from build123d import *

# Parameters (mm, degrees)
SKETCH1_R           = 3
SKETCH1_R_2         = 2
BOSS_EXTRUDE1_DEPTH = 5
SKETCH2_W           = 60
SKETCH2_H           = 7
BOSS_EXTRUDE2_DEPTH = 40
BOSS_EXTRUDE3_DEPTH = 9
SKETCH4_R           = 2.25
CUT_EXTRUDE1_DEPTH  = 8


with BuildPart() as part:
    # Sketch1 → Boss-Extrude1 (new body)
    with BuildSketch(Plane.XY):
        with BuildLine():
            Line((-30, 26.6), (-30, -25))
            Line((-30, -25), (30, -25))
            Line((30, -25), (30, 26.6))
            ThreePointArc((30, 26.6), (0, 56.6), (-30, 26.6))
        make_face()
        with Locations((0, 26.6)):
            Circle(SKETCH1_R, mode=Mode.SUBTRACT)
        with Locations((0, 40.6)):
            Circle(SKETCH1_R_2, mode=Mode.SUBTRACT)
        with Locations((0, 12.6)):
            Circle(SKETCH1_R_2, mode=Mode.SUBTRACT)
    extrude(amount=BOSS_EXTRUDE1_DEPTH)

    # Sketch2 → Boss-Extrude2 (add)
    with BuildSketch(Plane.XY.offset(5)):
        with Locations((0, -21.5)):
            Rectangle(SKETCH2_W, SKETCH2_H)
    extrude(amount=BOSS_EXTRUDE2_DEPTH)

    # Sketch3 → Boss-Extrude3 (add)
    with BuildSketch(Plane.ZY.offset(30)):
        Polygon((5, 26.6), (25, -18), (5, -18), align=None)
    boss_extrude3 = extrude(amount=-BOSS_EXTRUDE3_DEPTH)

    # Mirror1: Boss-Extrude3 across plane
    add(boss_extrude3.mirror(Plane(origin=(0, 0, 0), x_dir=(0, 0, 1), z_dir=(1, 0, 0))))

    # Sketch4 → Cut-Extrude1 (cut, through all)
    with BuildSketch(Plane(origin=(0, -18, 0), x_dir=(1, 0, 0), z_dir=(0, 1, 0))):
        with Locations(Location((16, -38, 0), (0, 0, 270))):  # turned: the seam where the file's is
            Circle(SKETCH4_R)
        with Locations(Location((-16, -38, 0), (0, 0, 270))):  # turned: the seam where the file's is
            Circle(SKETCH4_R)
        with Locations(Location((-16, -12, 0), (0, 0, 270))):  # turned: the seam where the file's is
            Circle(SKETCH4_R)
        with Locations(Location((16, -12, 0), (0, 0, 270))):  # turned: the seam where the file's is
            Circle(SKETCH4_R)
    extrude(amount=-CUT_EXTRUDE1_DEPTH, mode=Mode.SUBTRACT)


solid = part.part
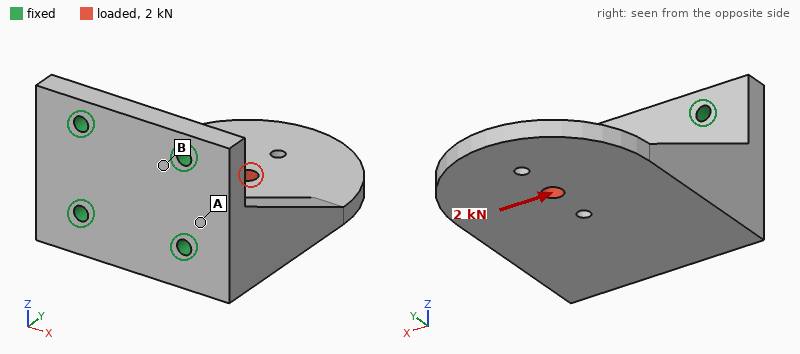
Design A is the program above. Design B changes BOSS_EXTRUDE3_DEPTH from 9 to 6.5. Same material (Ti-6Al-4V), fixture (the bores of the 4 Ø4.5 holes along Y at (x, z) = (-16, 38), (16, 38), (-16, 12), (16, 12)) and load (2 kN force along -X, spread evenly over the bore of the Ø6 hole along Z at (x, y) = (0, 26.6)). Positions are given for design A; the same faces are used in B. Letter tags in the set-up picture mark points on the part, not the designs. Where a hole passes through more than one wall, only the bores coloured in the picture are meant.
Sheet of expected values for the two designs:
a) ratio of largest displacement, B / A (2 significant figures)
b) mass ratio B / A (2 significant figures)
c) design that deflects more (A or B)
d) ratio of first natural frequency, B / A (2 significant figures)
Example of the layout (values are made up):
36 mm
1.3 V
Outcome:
1.1
0.95
B
0.91
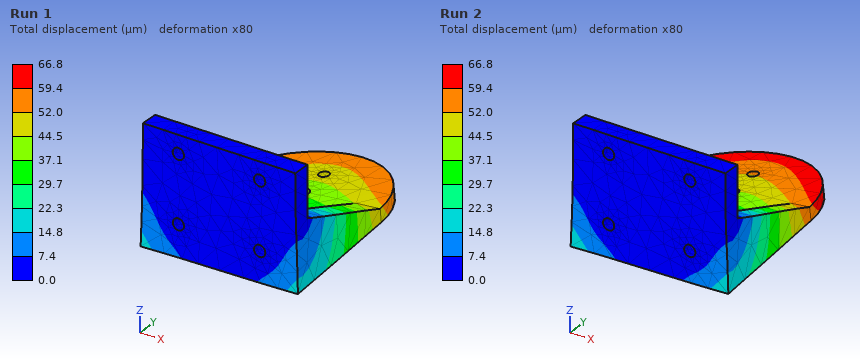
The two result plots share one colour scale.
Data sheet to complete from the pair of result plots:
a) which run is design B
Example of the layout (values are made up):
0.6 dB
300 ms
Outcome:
Run 2
